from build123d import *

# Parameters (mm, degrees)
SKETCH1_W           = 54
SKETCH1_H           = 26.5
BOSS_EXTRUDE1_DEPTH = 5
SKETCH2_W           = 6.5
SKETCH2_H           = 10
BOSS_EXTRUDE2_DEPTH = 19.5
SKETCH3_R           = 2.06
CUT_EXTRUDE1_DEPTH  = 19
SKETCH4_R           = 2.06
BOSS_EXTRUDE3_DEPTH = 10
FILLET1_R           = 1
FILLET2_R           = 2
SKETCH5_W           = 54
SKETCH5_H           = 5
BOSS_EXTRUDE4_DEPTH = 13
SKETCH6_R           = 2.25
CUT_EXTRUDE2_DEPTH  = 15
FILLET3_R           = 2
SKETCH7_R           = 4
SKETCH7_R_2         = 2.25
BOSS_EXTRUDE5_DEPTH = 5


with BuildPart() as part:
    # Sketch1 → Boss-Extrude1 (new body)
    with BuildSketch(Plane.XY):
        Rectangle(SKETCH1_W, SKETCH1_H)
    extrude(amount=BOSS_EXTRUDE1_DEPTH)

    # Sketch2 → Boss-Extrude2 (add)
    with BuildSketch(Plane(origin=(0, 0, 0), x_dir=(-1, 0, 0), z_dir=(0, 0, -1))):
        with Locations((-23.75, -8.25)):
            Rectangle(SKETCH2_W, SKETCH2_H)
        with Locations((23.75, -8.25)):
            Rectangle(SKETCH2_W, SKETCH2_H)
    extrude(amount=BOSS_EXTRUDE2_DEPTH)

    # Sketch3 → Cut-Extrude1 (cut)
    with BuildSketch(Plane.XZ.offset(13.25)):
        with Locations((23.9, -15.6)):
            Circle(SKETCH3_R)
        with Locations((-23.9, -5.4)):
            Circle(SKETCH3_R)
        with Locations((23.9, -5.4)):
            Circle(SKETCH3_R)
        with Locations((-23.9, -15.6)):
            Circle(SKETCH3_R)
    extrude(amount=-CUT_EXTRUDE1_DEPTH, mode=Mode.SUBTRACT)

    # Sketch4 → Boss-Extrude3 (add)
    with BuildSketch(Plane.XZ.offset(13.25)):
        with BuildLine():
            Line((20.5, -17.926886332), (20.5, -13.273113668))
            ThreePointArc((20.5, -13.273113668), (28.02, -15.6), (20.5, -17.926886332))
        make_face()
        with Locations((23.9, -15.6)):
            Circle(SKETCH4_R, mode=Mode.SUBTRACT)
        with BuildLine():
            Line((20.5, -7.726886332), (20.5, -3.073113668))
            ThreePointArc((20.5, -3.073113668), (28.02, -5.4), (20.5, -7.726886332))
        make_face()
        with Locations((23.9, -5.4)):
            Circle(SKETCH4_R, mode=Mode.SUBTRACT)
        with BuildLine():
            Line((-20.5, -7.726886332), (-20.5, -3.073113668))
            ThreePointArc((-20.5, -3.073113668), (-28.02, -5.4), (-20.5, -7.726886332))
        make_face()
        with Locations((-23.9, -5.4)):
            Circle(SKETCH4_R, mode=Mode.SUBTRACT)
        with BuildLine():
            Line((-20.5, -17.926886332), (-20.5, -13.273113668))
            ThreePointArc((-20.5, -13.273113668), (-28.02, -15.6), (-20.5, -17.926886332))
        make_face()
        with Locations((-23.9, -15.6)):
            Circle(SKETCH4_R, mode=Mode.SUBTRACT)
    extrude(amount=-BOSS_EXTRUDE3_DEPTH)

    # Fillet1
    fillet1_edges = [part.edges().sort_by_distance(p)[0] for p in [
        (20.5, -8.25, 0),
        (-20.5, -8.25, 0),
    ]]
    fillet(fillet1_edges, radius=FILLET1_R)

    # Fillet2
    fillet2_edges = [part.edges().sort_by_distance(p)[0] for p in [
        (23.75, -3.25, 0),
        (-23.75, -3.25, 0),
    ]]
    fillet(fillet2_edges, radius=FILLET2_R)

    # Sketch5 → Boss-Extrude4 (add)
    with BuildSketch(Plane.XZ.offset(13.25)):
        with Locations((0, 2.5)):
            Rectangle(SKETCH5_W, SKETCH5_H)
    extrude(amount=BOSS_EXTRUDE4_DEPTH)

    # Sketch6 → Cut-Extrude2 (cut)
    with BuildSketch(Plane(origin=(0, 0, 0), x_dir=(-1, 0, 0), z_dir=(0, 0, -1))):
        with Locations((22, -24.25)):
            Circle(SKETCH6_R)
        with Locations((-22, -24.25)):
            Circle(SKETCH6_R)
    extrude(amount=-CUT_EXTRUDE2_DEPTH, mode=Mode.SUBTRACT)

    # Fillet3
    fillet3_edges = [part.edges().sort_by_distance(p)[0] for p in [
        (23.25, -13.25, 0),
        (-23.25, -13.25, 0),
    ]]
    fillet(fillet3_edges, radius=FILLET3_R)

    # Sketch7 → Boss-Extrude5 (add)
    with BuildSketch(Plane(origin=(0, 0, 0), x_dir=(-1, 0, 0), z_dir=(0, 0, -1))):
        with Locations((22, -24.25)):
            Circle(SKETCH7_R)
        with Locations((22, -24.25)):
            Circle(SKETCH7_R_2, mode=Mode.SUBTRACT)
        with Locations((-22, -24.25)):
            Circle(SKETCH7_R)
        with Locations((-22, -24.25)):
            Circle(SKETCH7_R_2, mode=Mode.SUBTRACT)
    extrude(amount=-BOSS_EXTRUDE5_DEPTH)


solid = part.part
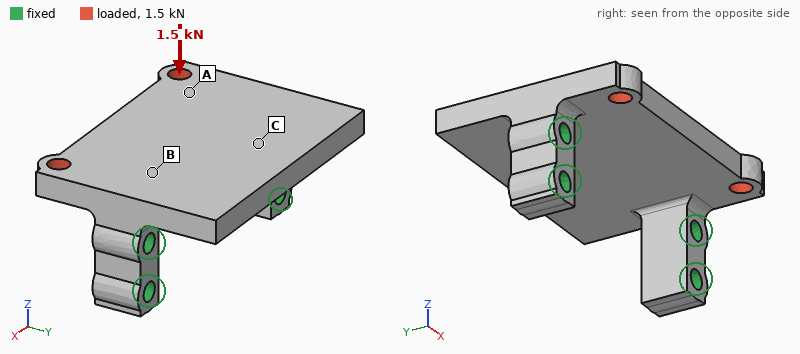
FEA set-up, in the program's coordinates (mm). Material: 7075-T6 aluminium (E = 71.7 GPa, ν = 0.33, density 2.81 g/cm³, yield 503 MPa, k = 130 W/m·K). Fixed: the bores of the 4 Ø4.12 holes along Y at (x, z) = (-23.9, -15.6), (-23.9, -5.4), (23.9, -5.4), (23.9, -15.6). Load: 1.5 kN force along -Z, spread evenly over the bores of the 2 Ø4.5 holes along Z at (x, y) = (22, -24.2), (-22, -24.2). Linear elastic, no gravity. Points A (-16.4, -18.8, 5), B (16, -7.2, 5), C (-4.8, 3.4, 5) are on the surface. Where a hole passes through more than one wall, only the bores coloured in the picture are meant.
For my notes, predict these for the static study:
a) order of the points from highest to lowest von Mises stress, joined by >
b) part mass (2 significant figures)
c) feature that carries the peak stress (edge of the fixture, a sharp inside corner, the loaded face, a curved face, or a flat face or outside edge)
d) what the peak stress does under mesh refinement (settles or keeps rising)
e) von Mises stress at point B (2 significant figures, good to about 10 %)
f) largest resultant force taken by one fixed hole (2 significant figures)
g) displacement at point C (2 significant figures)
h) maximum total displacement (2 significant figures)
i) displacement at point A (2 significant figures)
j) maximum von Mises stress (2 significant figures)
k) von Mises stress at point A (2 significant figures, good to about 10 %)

A > B > C
36 g
a curved face
settles
37 MPa
790 N
0.029 mm
0.11 mm
0.048 mm
410 MPa
55 MPa
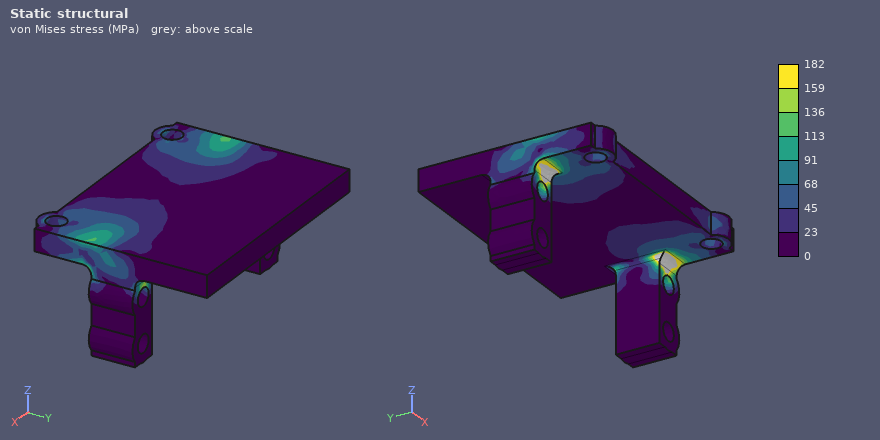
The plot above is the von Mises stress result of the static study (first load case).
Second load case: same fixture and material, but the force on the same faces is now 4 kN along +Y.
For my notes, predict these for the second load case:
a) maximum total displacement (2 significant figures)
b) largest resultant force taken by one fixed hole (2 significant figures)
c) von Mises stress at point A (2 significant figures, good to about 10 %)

43 µm
2.0 kN
20 MPa
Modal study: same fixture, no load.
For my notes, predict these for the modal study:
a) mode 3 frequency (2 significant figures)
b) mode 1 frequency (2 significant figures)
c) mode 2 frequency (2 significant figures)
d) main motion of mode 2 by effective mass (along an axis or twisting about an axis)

11 kHz
5800 Hz
7900 Hz
along Z
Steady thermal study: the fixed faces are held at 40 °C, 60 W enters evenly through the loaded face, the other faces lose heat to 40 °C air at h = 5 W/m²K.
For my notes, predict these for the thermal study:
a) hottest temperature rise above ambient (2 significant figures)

75 K
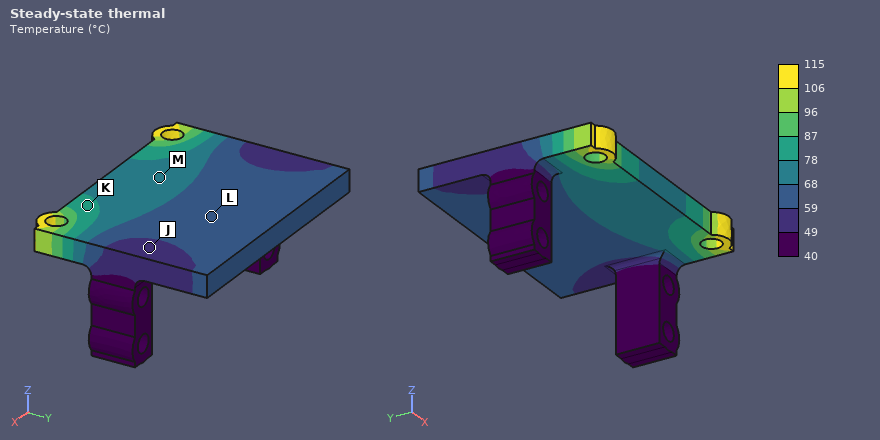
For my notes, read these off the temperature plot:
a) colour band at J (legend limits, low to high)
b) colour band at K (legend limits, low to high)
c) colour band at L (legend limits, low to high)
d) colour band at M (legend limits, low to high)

49 to 59 °C
78 to 87 °C
59 to 68 °C
68 to 78 °C
